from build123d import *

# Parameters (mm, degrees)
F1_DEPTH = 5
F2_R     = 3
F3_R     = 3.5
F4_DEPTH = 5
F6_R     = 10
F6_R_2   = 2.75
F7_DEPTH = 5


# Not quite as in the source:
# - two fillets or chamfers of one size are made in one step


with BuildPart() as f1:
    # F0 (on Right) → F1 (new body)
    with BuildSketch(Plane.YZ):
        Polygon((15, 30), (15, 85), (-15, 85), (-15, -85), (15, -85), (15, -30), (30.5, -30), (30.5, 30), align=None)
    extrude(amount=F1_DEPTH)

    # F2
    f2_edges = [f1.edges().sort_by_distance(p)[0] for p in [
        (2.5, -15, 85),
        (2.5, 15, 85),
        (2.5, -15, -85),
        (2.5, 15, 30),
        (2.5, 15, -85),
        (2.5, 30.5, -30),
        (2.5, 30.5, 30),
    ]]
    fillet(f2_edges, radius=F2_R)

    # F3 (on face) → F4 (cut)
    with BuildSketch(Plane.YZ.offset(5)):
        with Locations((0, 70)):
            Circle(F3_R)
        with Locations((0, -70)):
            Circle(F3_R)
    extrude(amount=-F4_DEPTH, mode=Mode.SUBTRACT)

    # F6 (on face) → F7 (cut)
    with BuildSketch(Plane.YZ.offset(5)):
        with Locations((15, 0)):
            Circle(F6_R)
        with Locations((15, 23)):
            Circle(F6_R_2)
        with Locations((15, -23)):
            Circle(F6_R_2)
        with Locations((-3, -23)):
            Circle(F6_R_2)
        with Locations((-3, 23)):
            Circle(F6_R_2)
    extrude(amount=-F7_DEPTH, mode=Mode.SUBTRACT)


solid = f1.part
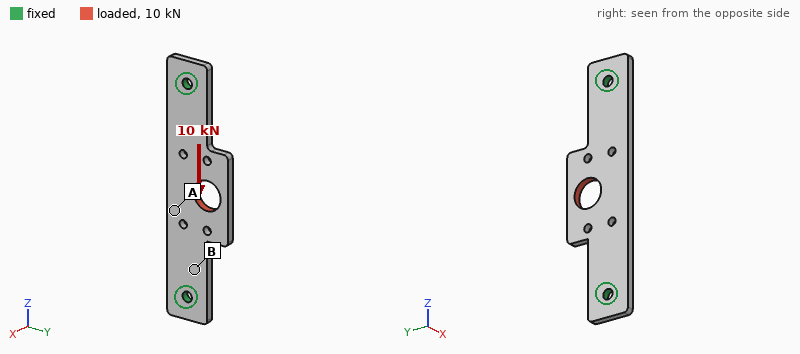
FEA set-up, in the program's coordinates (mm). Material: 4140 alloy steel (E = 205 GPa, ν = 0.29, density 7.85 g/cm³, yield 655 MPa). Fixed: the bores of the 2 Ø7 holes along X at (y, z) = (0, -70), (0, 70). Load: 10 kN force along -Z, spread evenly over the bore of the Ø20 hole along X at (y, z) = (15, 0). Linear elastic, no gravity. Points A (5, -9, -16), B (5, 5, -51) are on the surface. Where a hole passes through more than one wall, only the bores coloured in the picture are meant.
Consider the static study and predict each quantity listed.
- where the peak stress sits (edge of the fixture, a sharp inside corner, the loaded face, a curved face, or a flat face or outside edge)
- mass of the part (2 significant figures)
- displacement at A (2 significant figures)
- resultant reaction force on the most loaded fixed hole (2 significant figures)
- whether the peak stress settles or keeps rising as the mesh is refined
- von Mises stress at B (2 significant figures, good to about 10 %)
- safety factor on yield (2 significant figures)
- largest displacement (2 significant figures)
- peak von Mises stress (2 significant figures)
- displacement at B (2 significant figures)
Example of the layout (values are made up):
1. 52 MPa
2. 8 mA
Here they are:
1. a curved face
2. 220 g
3. 8.0 µm
4. 5.2 kN
5. settles
6. 48 MPa
7. 2.7
8. 25 µm
9. 240 MPa
10. 5.4 µm
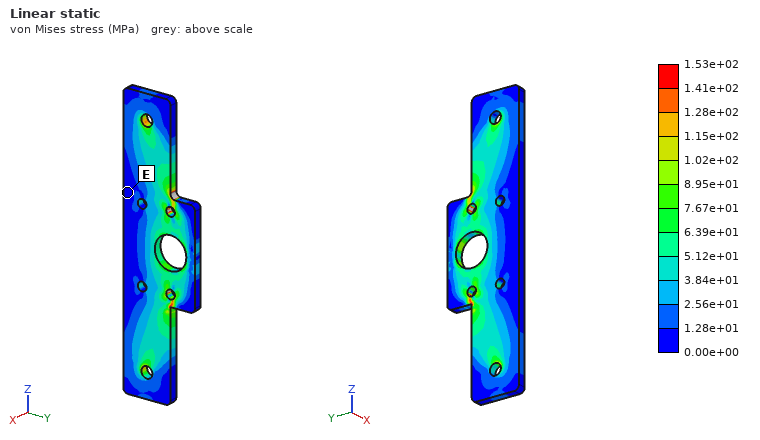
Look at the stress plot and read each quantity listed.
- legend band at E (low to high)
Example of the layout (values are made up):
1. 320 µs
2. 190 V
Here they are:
1. 0.00e+00 to 1.28e+01 MPa
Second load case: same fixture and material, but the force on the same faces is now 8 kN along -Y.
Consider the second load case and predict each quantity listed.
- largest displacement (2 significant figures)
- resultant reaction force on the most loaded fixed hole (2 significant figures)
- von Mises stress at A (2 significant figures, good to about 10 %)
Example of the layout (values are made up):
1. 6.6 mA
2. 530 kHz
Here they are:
1. 89 µm
2. 4.1 kN
3. 72 MPa
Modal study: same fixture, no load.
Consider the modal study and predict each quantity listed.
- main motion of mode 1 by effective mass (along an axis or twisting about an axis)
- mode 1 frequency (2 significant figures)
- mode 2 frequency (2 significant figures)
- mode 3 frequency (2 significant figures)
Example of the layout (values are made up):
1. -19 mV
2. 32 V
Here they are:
1. along X
2. 1200 Hz
3. 2300 Hz
4. 3300 Hz
